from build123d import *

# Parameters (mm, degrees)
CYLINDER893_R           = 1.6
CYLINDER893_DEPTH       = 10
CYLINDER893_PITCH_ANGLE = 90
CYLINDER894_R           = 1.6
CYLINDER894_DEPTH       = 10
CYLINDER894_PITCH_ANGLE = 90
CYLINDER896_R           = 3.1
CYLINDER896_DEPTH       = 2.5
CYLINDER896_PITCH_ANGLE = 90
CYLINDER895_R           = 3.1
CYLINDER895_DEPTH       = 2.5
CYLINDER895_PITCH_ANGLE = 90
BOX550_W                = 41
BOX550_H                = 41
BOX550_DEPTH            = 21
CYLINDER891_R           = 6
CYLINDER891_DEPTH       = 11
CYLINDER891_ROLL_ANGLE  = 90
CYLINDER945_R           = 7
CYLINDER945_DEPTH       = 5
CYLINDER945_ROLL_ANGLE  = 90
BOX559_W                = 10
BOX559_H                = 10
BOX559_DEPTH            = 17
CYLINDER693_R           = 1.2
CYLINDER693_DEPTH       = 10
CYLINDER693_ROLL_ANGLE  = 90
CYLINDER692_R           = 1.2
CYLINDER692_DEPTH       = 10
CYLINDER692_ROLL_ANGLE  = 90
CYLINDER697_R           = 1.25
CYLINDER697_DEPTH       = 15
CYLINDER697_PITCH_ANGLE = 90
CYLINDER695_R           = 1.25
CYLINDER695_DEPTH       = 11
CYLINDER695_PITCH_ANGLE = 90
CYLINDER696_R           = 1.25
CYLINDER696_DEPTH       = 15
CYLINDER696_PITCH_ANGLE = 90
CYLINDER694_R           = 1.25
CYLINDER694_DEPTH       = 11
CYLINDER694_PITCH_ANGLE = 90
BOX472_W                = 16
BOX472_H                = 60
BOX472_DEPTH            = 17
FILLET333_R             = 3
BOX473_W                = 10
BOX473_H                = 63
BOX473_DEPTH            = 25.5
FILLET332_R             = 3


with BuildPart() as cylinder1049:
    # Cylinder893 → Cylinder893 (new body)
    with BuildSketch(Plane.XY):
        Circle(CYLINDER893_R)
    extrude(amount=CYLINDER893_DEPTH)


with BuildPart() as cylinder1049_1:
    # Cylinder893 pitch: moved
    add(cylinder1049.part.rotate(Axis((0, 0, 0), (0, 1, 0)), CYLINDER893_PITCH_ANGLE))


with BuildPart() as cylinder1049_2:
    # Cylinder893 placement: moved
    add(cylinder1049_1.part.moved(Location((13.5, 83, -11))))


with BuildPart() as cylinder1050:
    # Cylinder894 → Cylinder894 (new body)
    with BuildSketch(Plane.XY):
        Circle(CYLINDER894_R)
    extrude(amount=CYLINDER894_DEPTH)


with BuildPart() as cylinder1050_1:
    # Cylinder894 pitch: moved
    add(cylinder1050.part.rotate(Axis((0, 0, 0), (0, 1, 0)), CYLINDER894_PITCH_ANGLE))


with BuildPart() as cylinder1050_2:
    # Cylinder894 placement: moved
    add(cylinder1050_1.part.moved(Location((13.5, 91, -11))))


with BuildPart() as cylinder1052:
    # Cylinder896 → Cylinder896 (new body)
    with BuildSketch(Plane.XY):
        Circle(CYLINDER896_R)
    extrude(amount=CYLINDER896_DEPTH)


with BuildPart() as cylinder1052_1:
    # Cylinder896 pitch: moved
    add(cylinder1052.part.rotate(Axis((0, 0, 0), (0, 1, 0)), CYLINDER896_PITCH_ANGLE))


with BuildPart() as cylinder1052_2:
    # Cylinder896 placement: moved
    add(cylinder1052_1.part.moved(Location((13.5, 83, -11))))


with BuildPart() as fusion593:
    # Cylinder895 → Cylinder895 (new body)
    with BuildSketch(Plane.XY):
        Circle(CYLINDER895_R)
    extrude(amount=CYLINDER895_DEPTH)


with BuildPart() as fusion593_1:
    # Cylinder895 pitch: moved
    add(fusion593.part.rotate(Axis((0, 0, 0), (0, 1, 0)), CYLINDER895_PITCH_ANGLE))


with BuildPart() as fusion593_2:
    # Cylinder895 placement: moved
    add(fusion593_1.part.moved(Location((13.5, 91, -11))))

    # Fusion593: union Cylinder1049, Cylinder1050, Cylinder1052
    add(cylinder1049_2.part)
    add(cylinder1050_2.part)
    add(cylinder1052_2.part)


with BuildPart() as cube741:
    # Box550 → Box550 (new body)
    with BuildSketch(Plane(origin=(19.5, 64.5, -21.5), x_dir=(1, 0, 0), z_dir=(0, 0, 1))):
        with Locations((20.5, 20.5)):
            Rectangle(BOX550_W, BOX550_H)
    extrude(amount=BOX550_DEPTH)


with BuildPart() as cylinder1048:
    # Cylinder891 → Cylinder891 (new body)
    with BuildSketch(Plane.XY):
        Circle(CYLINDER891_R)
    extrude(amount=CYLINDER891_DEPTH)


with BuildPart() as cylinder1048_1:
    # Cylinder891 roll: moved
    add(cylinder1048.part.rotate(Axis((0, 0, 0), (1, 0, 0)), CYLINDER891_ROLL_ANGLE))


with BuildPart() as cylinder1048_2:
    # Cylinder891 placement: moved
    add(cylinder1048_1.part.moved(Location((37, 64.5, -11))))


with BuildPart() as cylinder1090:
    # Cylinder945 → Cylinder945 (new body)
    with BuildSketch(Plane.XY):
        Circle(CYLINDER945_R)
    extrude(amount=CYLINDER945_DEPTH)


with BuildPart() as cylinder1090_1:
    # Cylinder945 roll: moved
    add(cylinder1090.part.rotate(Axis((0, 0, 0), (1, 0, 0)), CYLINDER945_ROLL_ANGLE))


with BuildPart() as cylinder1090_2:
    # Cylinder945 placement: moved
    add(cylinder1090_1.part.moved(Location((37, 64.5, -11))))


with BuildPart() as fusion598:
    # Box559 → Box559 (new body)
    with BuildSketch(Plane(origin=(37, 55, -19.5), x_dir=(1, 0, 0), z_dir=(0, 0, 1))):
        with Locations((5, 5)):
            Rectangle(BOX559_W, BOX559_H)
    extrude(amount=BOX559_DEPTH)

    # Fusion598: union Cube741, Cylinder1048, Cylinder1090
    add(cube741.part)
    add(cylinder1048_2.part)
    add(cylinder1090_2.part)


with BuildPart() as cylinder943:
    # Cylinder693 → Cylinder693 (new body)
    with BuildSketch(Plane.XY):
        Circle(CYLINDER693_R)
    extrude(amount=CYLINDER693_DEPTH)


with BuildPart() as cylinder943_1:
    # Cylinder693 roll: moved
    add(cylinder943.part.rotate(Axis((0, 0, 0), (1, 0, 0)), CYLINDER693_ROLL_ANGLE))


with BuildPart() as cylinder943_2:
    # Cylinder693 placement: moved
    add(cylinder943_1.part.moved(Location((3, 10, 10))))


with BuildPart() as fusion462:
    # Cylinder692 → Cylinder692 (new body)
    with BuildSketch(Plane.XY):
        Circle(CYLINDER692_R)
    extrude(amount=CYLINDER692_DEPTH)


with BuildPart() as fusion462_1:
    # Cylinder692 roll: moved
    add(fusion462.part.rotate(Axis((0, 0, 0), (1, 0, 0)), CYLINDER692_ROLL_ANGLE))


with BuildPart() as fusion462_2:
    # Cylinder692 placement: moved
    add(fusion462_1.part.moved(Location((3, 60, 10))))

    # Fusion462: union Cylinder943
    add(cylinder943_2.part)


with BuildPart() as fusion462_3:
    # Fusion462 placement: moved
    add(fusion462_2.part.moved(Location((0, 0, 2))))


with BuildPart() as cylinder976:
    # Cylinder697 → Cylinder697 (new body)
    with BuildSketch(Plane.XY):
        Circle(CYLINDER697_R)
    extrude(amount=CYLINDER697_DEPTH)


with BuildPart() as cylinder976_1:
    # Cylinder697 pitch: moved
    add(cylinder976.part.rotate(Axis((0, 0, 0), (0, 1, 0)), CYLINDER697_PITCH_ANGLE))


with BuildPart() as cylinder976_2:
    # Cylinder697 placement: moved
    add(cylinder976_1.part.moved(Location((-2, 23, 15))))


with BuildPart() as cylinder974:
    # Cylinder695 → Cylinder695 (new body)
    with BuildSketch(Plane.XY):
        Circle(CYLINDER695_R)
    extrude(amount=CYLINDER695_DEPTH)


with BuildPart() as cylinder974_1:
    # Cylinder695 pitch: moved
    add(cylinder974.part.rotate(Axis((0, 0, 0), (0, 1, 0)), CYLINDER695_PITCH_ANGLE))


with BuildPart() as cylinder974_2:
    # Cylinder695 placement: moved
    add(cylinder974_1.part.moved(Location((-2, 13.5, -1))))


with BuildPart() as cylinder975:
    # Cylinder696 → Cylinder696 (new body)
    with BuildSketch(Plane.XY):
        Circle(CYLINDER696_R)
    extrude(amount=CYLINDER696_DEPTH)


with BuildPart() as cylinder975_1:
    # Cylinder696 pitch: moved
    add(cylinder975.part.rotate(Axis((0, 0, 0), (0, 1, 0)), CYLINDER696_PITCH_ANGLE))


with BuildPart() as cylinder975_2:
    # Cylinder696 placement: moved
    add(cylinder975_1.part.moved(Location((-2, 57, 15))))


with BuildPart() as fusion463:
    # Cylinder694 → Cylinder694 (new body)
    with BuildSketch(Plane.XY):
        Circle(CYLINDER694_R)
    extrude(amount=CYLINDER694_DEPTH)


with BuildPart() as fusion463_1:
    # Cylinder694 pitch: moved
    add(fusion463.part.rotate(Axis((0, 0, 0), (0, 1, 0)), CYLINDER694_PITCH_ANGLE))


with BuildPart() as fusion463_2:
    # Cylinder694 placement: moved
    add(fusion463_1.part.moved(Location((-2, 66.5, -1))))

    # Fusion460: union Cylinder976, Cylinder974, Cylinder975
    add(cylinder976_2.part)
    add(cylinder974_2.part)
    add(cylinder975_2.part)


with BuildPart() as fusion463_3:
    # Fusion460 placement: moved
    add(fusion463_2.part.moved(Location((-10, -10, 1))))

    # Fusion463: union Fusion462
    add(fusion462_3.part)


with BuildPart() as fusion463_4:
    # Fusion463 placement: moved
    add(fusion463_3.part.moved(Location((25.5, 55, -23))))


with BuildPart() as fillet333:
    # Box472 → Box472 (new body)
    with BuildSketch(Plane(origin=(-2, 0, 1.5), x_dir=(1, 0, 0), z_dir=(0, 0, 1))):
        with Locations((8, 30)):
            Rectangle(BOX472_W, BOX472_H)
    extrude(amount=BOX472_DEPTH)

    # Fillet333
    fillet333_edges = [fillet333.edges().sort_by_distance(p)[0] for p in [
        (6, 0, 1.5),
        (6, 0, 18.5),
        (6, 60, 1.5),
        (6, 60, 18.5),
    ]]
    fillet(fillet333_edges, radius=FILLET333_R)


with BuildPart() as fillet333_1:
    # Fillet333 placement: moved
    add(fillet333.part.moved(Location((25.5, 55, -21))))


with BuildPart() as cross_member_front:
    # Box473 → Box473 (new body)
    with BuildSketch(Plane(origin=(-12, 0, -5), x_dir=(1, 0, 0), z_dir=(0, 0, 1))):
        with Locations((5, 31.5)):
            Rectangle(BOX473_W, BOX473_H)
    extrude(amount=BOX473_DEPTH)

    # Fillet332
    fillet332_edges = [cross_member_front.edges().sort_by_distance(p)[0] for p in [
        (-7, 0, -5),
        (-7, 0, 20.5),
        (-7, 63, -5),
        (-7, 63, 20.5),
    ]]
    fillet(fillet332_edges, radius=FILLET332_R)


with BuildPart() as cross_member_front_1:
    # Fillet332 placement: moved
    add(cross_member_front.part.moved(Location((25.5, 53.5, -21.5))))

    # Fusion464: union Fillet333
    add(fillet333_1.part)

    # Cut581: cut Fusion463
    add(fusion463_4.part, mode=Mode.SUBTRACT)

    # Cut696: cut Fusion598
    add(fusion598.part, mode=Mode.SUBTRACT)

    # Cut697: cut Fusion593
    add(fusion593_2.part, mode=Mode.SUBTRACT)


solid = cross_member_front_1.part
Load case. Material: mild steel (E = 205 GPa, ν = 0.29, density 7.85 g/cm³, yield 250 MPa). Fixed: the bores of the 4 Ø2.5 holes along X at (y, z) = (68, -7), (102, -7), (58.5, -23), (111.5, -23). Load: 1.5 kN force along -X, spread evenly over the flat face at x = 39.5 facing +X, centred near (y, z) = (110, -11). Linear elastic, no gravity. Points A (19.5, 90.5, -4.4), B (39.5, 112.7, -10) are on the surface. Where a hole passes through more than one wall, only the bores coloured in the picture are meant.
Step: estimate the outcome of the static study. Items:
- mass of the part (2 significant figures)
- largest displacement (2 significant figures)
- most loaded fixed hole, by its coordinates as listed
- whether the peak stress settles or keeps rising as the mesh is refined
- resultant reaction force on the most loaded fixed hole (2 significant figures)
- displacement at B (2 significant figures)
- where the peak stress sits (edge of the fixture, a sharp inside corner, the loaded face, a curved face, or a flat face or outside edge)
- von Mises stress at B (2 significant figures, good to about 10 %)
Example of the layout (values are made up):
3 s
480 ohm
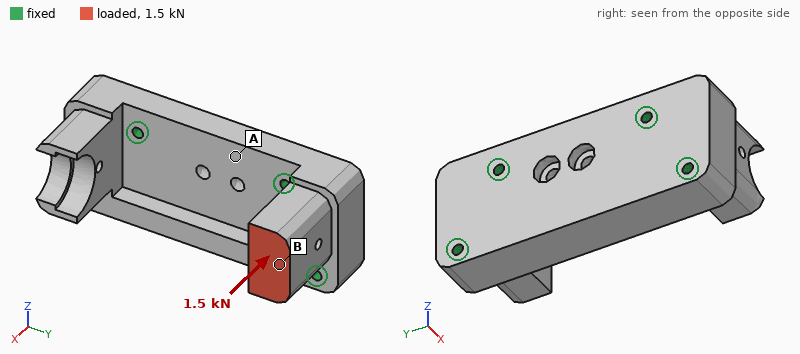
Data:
130 g
6.3 µm
(102, -7)
keeps rising
810 N
5.4 µm
edge of the fixture
9.2 MPa
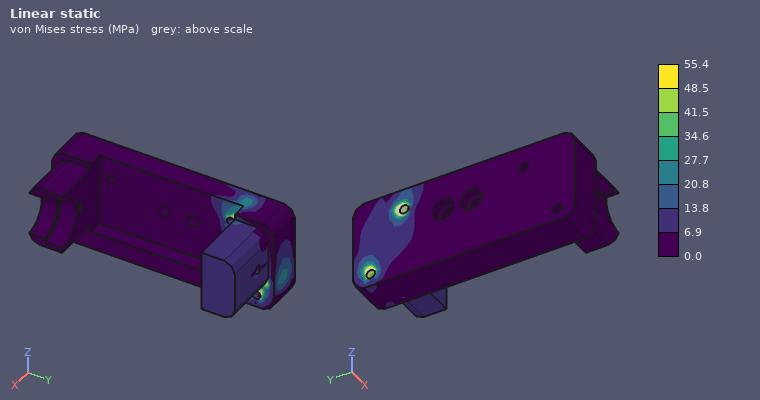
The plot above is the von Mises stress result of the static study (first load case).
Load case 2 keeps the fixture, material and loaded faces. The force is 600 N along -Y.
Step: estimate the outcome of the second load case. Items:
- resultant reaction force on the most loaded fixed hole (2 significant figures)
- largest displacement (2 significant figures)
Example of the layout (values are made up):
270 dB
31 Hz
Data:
480 N
17 µm
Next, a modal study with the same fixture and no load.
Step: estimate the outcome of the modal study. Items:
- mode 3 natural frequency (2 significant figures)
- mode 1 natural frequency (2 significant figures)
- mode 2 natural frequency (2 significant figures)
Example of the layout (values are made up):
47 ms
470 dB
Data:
17 kHz
10000 Hz
15 kHz
